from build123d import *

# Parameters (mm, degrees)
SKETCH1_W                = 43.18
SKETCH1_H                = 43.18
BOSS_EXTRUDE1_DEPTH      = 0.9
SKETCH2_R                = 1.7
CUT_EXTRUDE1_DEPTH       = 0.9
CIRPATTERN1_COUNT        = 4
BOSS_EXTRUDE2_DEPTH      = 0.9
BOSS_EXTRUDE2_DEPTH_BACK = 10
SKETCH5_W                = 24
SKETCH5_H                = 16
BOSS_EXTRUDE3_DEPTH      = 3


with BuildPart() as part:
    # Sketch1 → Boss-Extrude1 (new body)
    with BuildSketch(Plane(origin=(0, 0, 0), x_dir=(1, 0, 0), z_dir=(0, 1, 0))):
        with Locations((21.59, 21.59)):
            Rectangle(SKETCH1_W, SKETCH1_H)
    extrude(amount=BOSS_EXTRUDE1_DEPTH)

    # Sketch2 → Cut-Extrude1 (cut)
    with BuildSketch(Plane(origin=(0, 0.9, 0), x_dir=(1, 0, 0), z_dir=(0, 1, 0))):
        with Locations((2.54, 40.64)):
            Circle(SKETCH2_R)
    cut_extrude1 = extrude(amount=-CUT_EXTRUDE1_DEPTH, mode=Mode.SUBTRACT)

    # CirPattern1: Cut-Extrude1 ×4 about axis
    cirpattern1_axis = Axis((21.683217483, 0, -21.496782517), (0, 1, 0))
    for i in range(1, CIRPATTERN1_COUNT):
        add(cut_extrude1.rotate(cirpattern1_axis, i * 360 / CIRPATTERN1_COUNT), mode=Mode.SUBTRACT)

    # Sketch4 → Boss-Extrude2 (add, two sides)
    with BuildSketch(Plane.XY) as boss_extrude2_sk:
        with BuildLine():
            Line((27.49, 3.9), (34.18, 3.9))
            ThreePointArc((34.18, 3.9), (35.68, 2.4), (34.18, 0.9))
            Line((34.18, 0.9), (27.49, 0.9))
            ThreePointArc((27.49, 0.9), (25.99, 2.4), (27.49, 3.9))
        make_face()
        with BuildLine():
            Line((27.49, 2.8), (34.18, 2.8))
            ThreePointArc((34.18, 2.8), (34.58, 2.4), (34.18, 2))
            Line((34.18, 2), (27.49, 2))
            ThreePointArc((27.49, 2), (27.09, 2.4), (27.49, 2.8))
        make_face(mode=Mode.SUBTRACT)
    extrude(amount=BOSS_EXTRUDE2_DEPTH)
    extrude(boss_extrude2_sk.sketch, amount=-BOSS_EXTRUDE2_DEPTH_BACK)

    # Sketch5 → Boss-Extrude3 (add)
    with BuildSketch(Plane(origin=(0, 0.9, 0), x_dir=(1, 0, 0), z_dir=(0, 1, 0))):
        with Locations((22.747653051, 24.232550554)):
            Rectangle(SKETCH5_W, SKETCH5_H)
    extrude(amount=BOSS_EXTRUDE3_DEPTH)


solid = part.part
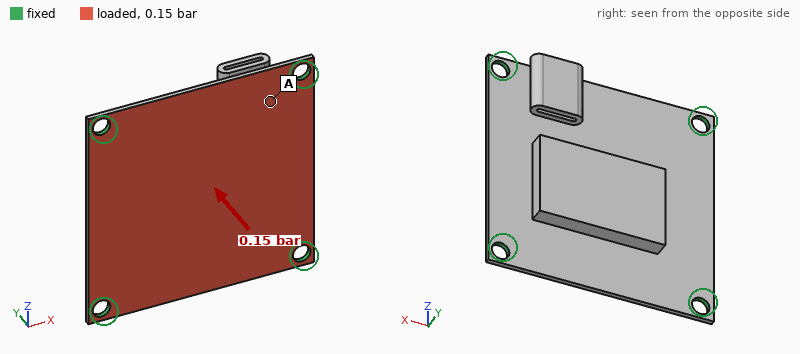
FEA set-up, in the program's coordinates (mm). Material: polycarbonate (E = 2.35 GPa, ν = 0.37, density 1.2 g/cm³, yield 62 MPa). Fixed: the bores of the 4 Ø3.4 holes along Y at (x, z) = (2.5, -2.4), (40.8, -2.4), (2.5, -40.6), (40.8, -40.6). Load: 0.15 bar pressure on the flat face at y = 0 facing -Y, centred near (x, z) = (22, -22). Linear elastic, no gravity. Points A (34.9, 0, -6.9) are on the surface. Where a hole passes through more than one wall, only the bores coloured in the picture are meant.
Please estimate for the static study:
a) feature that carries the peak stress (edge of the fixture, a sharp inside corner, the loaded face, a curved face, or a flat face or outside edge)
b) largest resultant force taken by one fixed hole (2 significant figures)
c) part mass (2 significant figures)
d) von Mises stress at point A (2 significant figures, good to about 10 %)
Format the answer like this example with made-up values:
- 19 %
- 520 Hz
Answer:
- the loaded face
- 8.0 N
- 3.6 g
- 3.2 MPa
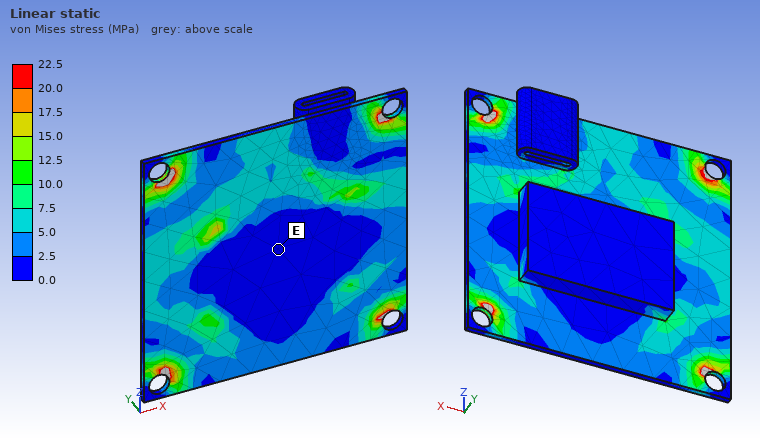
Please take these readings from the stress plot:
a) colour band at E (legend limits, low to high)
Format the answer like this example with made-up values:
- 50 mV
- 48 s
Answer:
- 0.0 to 2.5 MPa
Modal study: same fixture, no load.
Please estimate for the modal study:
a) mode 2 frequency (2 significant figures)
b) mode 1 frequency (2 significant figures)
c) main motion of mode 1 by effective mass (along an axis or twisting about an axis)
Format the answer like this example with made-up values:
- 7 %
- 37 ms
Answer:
- 1200 Hz
- 610 Hz
- along Y
